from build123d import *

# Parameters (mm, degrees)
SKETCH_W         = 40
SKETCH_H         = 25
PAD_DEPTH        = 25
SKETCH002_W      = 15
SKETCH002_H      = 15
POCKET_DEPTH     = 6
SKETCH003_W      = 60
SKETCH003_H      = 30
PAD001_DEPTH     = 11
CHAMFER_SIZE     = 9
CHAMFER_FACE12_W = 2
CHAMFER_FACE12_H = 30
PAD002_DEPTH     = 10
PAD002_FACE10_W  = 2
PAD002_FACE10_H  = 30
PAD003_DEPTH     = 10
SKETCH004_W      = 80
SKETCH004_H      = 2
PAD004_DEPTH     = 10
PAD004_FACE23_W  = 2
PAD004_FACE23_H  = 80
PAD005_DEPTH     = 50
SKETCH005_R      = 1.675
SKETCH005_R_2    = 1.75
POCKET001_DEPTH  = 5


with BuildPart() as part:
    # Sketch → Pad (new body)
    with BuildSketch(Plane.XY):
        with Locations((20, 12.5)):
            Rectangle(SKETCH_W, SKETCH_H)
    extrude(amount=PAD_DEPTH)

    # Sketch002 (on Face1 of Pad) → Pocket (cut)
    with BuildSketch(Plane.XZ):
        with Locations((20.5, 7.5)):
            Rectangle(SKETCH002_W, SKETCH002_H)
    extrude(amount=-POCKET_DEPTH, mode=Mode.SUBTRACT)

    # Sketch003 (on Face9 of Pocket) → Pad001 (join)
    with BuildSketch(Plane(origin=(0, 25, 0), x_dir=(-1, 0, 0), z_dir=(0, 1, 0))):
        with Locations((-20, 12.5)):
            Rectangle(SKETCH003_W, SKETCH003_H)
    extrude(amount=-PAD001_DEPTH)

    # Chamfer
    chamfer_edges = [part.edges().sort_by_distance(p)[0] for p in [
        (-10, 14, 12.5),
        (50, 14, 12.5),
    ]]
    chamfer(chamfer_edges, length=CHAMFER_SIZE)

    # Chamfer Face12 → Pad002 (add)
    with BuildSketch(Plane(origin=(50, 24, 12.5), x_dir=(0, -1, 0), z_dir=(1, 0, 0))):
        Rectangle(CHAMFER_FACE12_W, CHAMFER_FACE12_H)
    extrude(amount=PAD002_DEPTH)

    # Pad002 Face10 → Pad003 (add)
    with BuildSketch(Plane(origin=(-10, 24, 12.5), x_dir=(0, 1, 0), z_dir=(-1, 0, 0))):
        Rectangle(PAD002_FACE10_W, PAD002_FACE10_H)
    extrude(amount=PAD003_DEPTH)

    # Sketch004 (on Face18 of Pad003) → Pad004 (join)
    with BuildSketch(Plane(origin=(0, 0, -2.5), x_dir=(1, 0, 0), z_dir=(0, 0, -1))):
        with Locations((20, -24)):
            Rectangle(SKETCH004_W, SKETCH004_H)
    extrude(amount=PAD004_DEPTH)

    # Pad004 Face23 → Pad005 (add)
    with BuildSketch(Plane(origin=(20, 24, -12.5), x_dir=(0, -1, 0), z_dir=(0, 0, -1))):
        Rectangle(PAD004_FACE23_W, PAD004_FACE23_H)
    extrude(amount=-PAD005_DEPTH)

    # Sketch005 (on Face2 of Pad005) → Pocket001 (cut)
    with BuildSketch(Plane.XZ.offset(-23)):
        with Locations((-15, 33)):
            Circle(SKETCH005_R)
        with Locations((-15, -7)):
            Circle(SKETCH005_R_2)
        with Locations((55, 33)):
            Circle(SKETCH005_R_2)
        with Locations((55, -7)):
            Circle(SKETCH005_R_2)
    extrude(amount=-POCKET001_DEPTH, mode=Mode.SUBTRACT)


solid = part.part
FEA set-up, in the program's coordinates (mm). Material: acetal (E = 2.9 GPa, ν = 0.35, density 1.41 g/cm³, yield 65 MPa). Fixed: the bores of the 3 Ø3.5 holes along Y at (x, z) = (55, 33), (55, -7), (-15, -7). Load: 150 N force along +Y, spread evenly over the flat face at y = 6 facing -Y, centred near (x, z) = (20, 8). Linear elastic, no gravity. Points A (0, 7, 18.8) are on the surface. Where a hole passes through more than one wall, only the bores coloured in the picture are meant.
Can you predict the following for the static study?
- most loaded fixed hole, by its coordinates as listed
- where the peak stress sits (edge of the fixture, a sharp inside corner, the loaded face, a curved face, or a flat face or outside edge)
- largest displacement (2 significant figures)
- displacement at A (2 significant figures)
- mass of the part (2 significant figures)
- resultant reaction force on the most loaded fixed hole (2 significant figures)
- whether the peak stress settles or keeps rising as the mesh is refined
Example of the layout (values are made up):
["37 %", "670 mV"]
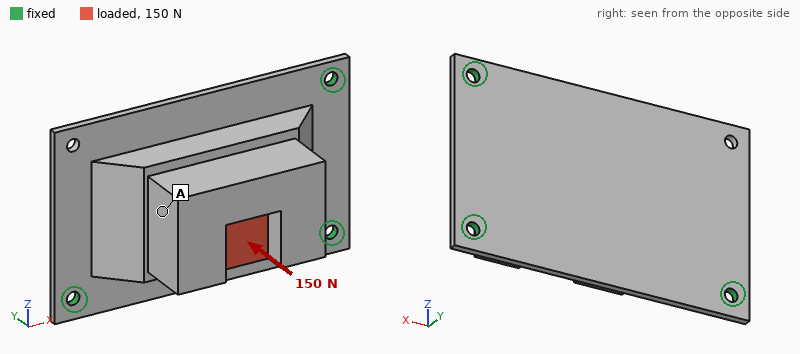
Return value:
["(-15, -7)", "edge of the fixture", "0.39 mm", "0.28 mm", "48 g", "96 N", "keeps rising"]
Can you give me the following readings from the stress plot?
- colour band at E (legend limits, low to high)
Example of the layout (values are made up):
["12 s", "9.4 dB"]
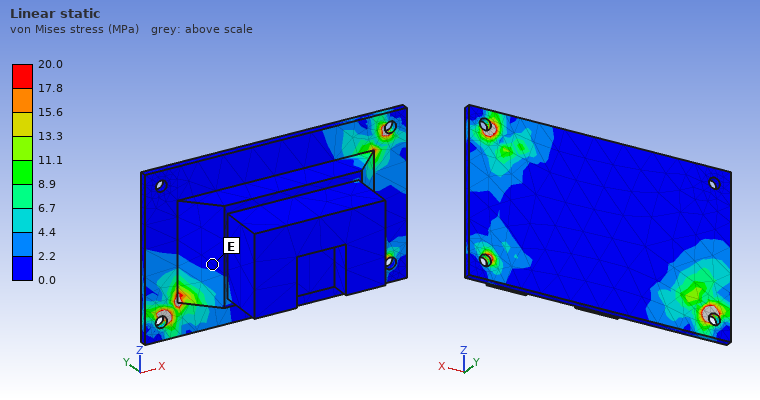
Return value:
["0.0 to 2.2 MPa"]
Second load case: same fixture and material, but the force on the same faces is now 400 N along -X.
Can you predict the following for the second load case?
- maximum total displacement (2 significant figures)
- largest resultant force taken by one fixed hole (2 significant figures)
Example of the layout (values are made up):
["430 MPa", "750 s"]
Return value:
["0.86 mm", "220 N"]
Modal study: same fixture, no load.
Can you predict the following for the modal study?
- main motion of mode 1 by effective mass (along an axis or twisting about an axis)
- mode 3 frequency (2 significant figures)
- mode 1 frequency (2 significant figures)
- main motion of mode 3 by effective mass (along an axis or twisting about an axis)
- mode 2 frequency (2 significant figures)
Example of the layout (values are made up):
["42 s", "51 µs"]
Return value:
["along Y", "1200 Hz", "470 Hz", "along X", "910 Hz"]
